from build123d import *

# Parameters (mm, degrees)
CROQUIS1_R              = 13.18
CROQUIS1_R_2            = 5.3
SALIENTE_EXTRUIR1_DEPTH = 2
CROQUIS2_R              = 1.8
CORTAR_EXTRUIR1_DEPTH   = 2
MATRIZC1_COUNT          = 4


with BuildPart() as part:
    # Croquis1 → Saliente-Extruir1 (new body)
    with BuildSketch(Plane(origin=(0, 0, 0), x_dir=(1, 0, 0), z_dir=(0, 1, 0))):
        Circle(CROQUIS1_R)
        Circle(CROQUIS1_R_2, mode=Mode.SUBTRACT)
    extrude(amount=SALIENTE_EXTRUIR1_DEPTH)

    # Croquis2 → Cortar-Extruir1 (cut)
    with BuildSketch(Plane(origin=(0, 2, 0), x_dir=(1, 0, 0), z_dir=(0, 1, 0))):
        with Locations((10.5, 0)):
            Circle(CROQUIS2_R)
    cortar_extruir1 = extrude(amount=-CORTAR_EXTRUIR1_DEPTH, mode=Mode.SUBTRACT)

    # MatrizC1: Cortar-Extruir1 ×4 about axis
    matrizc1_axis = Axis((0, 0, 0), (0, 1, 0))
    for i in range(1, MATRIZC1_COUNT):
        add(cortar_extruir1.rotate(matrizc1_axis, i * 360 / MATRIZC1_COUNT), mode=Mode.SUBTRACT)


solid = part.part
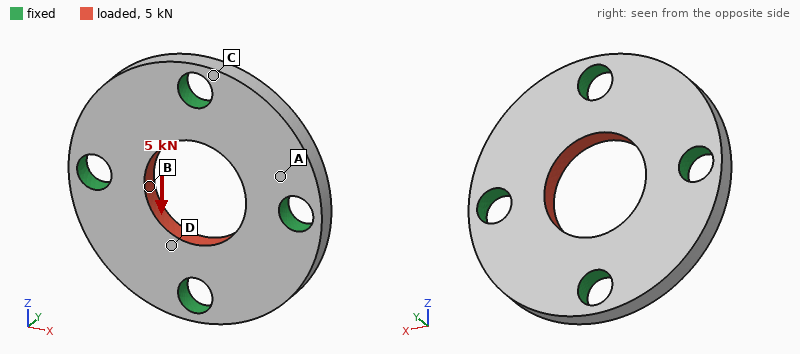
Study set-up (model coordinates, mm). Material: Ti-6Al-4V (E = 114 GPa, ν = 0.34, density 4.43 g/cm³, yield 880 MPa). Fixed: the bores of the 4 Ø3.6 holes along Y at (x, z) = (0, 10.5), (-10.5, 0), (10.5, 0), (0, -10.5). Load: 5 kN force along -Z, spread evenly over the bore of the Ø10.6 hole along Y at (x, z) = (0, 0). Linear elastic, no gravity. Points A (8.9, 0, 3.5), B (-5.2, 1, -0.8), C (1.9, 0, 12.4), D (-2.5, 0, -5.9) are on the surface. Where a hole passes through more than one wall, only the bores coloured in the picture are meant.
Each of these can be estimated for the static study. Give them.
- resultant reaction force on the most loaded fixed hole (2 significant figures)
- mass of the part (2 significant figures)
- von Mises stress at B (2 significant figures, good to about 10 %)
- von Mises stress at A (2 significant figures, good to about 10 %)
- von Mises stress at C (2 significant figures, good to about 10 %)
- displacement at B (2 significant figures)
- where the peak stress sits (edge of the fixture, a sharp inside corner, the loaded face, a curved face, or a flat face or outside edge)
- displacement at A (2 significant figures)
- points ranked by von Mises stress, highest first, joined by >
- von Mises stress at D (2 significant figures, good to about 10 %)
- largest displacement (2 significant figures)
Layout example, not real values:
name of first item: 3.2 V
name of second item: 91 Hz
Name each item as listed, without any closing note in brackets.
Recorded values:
resultant reaction force on the most loaded fixed hole: 1.4 kN
mass of the part: 3.7 g
von Mises stress at B: 130 MPa
von Mises stress at A: 55 MPa
von Mises stress at C: 24 MPa
displacement at B: 6.4 µm
where the peak stress sits: edge of the fixture
displacement at A: 2.2 µm
points ranked by von Mises stress, highest first, joined by >: B > D > A > C
von Mises stress at D: 100 MPa
largest displacement: 6.4 µm
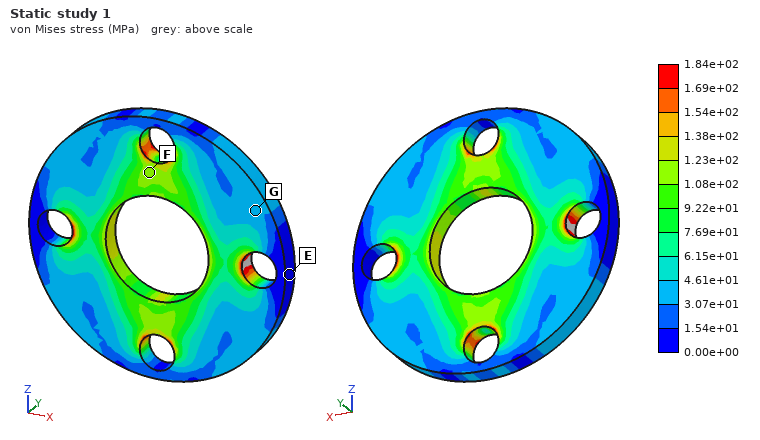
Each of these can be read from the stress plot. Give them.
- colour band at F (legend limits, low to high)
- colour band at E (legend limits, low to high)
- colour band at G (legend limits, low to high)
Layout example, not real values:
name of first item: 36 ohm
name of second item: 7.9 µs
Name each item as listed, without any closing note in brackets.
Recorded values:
colour band at F: 1.08e+02 to 1.23e+02 MPa
colour band at E: 0.00e+00 to 1.54e+01 MPa
colour band at G: 3.07e+01 to 4.61e+01 MPa
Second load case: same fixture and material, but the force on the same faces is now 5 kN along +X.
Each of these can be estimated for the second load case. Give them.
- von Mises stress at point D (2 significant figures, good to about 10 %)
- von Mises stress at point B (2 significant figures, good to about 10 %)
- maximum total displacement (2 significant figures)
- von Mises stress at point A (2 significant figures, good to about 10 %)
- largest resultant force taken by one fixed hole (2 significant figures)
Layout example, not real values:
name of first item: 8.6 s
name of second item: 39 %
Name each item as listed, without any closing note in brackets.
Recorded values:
von Mises stress at point D: 66 MPa
von Mises stress at point B: 120 MPa
maximum total displacement: 6.4 µm
von Mises stress at point A: 57 MPa
largest resultant force taken by one fixed hole: 1.4 kN
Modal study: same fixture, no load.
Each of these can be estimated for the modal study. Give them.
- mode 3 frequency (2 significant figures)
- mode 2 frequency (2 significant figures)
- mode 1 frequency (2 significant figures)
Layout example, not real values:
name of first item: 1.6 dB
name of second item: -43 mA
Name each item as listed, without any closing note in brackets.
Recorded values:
mode 3 frequency: 45 kHz
mode 2 frequency: 45 kHz
mode 1 frequency: 45 kHz
